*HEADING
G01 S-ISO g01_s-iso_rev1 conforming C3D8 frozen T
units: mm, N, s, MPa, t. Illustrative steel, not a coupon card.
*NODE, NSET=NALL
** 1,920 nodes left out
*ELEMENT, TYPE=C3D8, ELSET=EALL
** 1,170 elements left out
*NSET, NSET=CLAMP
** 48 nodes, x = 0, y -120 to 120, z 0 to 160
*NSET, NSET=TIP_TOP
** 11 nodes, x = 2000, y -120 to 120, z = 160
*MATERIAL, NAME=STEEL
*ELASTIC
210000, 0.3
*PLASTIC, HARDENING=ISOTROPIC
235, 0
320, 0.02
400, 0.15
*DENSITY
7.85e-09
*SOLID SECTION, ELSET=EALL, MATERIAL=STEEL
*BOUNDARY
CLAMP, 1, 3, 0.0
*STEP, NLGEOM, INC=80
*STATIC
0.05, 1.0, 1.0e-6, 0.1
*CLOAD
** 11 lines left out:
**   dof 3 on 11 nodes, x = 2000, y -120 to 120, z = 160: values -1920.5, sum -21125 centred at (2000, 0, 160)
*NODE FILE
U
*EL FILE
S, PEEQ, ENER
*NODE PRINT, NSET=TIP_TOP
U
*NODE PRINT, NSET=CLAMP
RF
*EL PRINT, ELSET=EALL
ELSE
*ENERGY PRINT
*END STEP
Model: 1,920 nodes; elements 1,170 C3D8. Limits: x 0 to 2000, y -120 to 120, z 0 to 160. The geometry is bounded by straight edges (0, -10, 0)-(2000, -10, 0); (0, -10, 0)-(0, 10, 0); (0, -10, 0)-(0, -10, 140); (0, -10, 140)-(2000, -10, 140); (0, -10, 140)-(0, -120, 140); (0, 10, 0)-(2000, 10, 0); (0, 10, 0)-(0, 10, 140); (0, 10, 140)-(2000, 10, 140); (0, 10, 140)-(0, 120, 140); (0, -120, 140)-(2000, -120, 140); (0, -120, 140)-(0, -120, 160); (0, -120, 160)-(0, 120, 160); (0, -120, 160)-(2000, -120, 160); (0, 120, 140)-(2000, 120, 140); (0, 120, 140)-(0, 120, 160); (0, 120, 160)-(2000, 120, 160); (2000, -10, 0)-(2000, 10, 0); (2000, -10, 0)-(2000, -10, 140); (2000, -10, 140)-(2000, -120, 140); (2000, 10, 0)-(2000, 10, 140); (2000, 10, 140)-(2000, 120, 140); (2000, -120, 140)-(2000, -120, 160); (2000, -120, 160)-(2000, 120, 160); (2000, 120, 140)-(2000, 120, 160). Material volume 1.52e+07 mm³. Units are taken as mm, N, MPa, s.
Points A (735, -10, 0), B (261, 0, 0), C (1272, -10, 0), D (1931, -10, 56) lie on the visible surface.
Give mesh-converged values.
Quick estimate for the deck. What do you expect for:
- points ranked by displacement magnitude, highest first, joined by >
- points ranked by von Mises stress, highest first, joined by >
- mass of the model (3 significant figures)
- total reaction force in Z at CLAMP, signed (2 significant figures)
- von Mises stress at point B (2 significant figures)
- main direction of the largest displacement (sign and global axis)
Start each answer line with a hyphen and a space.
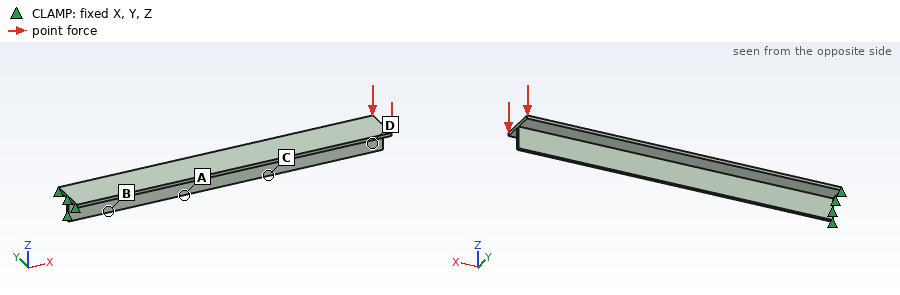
- D > C > A > B
- B > A > C > D
- 119 kg
- 21000 N
- 240 MPa
- -Z
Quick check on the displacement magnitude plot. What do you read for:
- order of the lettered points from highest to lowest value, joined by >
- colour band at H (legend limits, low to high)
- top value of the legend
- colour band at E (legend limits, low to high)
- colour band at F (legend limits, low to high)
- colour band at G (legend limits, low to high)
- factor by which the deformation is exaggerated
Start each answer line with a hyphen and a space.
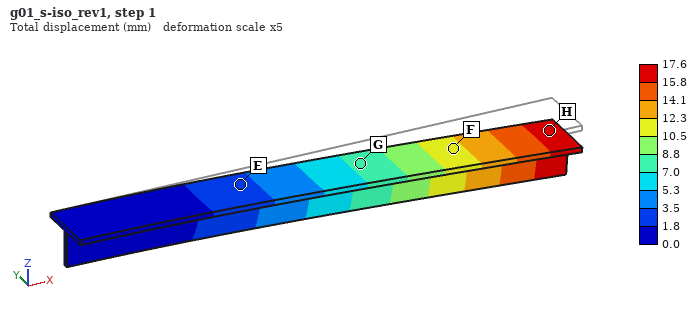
- H > F > G > E
- 15.8 to 17.6 mm
- 17.6 mm
- 1.8 to 3.5 mm
- 10.5 to 12.3 mm
- 7.0 to 8.8 mm
- 5
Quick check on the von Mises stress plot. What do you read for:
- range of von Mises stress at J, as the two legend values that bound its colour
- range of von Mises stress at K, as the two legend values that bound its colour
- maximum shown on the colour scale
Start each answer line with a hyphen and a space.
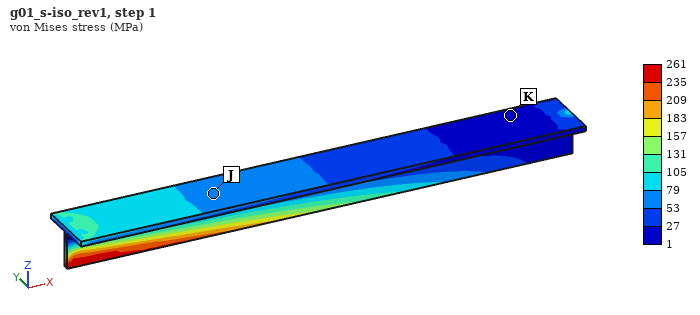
- 53 to 79 MPa
- 1 to 27 MPa
- 261 MPa
